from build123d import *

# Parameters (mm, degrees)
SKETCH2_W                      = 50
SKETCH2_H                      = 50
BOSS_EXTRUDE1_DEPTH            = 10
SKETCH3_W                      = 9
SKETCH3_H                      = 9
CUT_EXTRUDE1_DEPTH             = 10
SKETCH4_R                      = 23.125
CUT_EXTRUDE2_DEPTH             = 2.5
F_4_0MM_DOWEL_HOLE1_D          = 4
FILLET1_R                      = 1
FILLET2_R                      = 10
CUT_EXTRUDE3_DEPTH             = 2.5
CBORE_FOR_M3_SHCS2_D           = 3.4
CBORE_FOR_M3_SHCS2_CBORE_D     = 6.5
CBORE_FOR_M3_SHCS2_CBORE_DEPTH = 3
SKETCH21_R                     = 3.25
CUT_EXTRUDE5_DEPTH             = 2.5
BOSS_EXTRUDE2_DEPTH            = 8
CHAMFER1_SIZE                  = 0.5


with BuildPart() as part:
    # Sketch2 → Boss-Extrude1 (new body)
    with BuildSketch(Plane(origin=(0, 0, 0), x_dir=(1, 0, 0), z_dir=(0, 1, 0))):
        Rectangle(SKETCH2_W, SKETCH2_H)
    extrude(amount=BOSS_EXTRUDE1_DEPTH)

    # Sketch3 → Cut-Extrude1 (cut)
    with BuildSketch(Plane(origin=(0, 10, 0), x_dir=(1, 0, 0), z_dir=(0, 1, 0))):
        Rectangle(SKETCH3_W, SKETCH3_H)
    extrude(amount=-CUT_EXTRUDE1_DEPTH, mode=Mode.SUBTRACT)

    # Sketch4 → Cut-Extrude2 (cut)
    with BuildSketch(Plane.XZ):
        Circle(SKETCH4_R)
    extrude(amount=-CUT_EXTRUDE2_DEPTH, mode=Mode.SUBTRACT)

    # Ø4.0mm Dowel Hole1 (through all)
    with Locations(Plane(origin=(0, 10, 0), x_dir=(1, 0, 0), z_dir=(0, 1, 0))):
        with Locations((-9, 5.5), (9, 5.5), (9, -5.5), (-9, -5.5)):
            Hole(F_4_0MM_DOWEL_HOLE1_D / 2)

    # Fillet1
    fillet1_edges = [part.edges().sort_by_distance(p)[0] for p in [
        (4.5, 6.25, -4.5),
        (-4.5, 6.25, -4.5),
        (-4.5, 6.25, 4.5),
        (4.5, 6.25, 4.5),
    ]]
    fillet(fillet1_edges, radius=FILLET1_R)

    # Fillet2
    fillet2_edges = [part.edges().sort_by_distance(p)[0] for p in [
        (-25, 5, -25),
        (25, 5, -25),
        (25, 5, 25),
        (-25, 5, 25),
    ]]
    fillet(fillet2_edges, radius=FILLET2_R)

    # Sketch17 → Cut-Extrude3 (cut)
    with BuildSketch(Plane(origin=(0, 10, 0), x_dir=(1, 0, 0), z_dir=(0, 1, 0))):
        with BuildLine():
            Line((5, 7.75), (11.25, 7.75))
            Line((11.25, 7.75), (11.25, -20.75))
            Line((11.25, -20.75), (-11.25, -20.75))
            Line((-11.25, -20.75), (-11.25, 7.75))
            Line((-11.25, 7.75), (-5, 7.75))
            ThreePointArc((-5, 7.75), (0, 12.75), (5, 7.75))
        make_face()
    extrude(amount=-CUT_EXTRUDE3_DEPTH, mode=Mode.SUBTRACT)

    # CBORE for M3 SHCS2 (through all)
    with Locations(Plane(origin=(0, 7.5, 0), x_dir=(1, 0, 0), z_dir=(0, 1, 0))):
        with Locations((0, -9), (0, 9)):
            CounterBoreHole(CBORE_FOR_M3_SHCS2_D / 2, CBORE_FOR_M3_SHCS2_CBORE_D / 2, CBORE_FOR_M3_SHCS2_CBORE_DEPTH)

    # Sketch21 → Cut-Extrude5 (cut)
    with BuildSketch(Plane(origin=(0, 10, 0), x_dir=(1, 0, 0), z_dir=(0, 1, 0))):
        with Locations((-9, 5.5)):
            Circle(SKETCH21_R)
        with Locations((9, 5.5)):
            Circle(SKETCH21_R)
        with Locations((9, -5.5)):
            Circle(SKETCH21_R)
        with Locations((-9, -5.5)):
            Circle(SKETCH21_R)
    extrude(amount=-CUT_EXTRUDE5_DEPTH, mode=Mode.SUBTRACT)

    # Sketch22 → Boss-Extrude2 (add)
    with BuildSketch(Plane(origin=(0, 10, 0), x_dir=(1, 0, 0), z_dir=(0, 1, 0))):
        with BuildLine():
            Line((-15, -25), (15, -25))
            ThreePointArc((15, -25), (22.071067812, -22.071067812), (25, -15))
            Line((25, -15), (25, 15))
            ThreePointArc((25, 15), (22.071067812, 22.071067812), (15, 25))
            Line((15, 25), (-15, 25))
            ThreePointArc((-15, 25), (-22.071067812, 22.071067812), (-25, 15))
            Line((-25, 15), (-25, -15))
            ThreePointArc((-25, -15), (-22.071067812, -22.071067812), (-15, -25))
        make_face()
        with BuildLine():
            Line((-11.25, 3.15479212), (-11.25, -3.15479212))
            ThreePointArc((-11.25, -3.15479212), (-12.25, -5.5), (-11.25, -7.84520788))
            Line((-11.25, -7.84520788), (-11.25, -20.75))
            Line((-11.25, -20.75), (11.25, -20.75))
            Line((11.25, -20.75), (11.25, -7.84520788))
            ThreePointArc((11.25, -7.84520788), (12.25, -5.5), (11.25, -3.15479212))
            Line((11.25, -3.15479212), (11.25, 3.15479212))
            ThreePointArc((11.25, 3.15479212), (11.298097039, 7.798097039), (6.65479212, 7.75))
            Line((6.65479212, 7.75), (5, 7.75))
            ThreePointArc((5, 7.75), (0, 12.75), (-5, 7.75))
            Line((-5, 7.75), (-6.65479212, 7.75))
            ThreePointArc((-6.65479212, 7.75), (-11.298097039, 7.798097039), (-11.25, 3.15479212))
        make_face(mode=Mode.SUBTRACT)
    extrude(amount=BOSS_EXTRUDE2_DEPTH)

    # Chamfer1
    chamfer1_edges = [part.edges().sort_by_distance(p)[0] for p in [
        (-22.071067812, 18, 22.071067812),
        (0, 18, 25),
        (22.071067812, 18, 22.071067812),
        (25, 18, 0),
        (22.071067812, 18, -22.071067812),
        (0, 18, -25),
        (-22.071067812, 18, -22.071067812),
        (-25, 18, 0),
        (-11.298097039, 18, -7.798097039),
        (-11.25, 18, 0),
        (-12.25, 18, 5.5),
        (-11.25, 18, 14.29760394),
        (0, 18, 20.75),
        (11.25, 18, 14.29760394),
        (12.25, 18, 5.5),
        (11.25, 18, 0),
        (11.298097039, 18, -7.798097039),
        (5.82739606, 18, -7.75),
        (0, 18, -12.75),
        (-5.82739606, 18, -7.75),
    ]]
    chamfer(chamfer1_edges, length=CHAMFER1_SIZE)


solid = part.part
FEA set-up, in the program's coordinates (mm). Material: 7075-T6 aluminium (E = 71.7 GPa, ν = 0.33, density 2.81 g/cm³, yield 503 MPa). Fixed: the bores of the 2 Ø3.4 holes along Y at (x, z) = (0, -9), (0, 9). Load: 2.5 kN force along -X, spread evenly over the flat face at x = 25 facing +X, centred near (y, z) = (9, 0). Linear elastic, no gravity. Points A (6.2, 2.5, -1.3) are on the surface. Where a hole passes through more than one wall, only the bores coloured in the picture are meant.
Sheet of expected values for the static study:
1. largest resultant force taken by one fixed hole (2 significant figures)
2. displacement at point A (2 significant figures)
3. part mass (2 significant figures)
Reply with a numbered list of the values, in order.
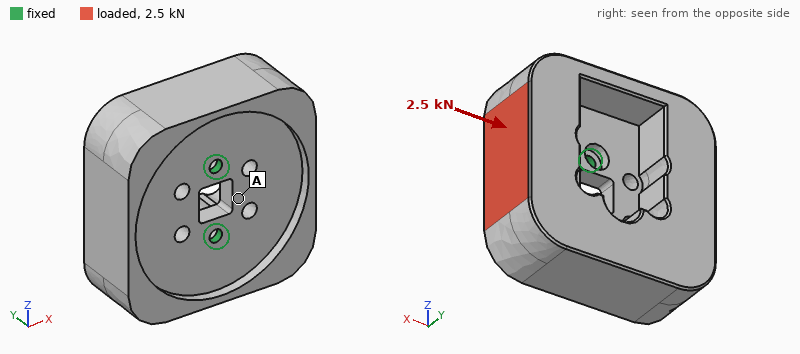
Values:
1. 1.3 kN
2. 0.041 mm
3. 87 g
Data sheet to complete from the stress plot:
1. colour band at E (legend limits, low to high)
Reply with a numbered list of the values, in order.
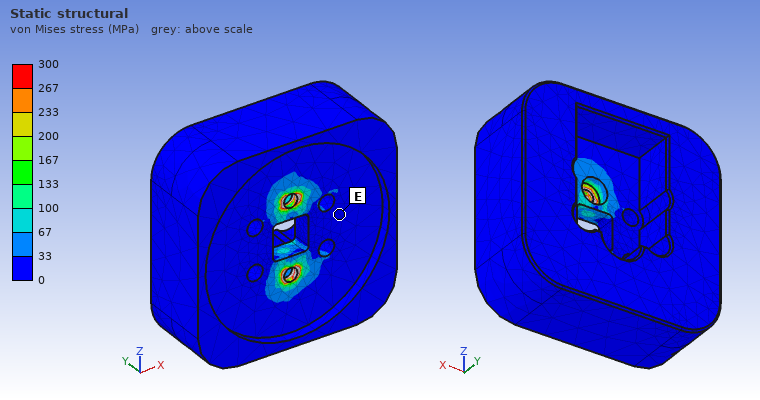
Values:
1. 0 to 33 MPa
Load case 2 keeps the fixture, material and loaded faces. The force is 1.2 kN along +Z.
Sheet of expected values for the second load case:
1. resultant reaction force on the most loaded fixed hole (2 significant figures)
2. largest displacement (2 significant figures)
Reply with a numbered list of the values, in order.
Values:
1. 1.6 kN
2. 29 µm
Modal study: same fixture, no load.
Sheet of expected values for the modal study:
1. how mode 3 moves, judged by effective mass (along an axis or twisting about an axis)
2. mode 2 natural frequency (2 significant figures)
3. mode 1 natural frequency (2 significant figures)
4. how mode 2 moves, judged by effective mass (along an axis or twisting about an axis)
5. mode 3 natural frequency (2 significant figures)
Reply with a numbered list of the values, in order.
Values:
1. twisting about Y
2. 4100 Hz
3. 1300 Hz
4. along Z
5. 5300 Hz
